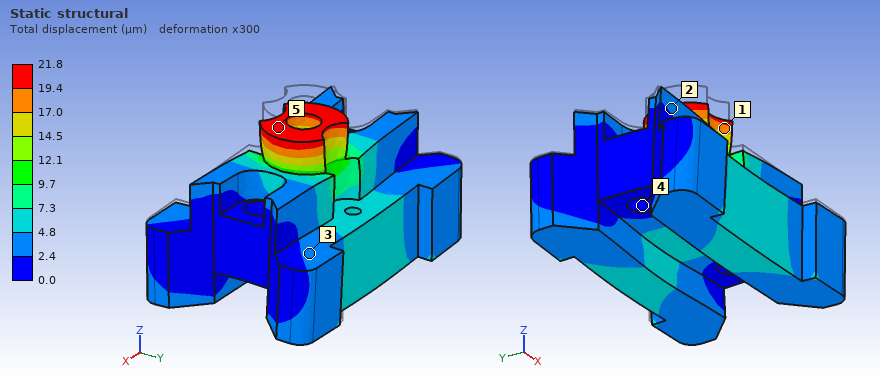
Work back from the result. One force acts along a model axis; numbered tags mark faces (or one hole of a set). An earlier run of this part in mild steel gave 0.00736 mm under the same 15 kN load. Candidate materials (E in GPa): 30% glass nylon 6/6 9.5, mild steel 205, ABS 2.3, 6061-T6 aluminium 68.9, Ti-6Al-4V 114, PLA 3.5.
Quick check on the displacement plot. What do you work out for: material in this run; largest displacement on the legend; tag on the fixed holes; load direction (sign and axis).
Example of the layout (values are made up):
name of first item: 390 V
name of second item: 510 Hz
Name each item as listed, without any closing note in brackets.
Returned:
material in this run: 6061-T6 aluminium
largest displacement on the legend: 21.8 µm
tag on the fixed holes: 4
load direction: -Z
